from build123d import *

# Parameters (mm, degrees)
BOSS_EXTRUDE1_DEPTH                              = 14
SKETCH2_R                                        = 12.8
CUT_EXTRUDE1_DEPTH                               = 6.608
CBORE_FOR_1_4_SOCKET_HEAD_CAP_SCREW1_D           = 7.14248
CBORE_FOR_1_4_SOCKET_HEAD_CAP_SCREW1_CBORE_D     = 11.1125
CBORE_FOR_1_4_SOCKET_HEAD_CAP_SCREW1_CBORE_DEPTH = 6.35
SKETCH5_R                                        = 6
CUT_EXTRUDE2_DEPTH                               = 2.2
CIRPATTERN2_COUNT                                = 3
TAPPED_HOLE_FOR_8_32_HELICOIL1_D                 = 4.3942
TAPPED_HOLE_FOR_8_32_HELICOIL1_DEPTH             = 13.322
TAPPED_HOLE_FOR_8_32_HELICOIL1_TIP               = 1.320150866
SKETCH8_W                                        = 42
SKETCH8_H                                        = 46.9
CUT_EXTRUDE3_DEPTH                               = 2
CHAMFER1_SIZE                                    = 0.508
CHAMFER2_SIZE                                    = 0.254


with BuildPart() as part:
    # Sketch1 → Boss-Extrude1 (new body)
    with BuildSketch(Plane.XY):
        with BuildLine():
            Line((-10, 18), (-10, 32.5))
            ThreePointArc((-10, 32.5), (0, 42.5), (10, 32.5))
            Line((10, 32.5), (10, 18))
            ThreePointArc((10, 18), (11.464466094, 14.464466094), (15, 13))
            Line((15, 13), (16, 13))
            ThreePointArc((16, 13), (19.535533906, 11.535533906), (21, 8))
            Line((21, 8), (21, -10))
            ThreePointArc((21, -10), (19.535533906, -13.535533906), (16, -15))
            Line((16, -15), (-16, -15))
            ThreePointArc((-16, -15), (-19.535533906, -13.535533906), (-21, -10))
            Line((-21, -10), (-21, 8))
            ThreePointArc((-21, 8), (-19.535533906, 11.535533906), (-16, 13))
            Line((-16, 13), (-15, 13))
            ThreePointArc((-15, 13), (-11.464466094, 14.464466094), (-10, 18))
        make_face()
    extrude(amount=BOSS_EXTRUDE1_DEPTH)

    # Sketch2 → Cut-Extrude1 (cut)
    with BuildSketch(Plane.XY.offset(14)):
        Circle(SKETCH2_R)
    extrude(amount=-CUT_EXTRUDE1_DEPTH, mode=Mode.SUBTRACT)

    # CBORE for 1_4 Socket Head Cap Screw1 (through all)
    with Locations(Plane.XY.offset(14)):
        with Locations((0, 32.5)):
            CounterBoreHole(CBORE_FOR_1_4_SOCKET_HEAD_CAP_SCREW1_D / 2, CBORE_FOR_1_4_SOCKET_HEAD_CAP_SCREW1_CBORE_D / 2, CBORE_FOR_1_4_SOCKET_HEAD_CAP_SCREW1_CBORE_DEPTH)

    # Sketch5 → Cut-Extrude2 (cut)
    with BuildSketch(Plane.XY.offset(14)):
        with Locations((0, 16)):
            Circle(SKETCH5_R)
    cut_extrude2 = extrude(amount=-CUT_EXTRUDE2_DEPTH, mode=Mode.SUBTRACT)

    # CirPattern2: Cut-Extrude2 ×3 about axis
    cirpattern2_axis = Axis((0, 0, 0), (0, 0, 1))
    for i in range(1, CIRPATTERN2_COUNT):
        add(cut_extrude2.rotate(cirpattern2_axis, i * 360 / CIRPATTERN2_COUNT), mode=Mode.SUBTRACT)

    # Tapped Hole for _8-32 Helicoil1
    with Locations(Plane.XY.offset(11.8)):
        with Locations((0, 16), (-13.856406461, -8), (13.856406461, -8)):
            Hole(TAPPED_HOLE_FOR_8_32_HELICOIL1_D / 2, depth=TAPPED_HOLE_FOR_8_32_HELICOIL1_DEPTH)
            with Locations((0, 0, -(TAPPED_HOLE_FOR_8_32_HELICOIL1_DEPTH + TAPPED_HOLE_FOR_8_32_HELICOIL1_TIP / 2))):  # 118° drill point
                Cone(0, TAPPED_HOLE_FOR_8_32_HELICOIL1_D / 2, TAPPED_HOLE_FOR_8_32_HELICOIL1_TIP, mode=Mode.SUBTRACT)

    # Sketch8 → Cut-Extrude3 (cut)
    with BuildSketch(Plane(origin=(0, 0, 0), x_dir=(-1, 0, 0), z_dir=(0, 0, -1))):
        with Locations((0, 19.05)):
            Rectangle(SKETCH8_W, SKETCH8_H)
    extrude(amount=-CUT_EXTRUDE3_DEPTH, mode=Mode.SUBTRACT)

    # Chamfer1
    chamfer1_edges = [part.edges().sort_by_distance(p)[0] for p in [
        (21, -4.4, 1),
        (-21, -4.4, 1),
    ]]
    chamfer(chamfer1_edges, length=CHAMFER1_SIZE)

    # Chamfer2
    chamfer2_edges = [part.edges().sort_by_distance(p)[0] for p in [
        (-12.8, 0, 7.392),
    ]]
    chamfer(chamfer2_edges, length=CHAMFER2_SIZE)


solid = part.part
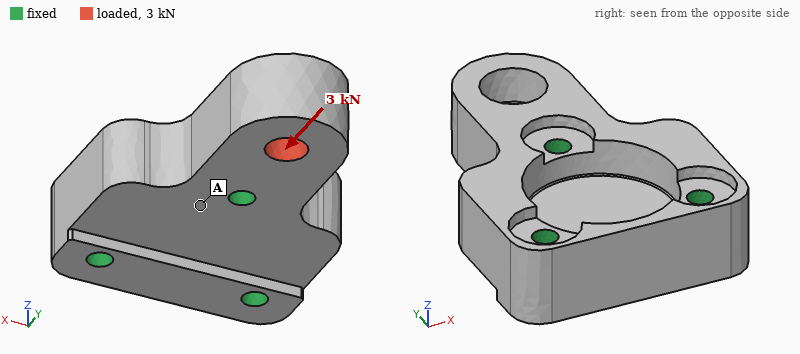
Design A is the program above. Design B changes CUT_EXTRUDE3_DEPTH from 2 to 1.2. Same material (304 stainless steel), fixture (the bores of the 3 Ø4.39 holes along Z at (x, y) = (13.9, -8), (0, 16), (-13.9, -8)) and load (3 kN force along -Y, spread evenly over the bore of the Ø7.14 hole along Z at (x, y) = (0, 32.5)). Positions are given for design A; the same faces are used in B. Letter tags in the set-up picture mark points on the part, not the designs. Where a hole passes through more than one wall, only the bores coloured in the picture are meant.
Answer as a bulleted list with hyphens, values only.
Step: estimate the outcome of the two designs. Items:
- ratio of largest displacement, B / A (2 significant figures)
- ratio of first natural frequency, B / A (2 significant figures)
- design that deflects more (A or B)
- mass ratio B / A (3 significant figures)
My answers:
- 0.84
- 1.1
- A
- 1.06
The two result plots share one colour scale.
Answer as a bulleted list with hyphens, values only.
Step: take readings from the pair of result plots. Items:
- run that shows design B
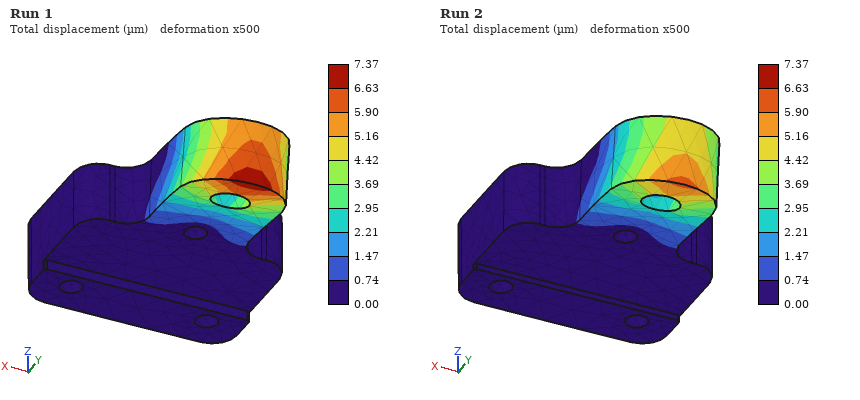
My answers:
- Run 2
